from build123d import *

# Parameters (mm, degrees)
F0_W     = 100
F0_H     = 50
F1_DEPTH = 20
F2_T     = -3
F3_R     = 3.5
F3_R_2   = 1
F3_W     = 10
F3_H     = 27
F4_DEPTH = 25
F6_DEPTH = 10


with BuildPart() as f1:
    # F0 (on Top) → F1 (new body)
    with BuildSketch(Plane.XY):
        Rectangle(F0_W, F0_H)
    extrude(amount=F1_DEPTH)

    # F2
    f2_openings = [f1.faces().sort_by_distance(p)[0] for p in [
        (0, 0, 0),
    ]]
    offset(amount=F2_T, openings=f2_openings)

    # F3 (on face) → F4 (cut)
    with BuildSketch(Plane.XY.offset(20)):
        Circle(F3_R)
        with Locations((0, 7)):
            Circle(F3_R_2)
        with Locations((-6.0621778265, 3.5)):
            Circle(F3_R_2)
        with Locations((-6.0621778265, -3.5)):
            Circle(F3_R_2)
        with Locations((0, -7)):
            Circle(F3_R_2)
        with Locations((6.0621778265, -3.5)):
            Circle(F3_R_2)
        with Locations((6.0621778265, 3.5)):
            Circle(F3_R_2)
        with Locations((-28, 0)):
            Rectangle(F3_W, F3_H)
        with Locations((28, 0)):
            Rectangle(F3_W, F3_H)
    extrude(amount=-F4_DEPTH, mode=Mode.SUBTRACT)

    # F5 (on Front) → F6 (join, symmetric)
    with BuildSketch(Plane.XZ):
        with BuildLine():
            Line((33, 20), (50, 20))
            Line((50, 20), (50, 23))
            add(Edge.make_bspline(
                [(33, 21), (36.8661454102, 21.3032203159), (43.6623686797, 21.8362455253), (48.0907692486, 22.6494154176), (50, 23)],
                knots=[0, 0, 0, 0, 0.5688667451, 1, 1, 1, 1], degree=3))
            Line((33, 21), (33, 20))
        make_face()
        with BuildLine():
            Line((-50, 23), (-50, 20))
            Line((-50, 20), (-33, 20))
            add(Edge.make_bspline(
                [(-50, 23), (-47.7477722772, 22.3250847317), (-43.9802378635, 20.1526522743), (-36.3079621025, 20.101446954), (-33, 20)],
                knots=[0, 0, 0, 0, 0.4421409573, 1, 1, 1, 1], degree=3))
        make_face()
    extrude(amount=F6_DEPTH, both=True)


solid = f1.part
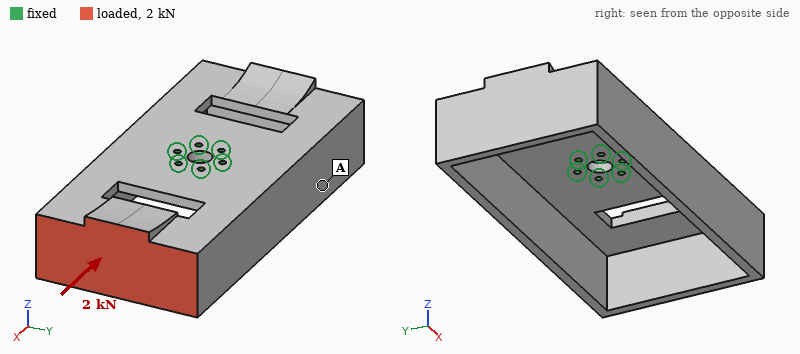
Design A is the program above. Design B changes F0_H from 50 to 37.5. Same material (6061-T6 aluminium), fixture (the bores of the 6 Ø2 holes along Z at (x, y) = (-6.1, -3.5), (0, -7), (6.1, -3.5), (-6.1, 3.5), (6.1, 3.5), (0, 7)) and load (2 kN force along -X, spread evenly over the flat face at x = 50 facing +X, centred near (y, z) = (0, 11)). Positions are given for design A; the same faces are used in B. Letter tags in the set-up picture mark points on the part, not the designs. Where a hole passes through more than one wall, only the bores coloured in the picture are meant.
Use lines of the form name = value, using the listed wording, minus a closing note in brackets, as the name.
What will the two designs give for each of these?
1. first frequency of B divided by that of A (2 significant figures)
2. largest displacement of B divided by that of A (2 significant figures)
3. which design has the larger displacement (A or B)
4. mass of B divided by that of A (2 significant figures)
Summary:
first frequency of B divided by that of A = 1.3
largest displacement of B divided by that of A = 0.65
which design has the larger displacement = A
mass of B divided by that of A = 0.83
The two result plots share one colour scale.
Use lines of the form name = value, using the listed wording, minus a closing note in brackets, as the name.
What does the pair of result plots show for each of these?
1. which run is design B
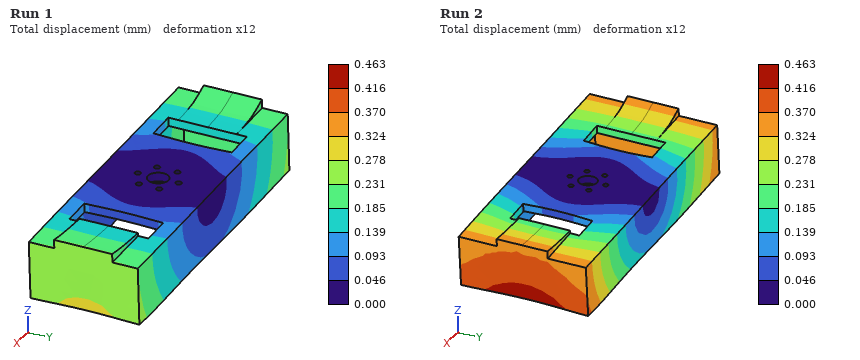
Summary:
which run is design B = Run 1
